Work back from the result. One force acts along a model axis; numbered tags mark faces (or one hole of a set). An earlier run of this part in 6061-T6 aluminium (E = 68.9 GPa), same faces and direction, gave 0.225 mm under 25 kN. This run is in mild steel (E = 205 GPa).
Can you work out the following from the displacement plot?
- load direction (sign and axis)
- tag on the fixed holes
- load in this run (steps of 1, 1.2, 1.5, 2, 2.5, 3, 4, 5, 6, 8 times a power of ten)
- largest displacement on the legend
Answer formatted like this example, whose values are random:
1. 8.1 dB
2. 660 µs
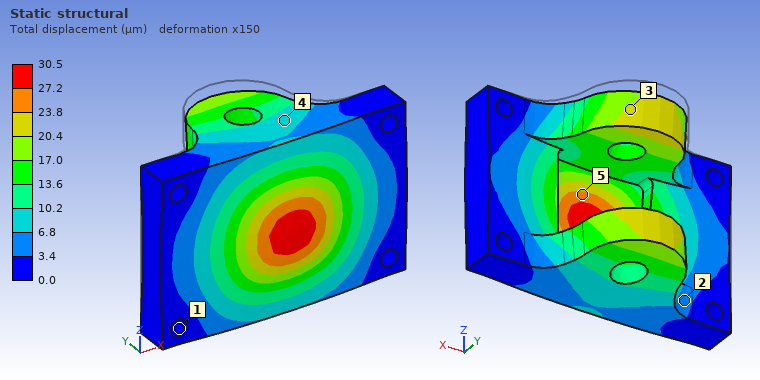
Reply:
1. -Y
2. 1
3. 10 kN
4. 30.5 µm
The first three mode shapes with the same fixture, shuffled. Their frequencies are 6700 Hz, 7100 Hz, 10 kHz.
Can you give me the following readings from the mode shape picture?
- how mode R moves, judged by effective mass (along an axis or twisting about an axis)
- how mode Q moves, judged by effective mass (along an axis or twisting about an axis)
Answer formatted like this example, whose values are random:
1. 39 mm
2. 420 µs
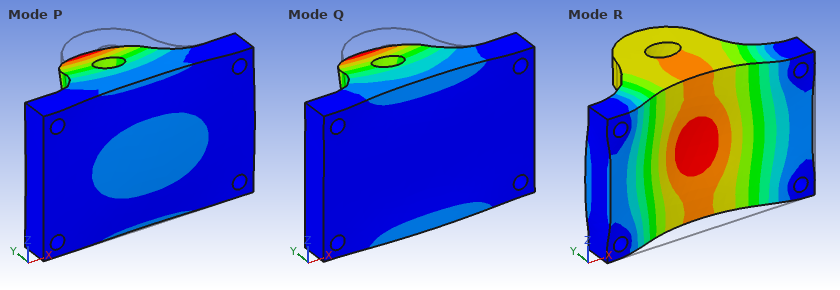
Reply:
1. along Y
2. along Z
